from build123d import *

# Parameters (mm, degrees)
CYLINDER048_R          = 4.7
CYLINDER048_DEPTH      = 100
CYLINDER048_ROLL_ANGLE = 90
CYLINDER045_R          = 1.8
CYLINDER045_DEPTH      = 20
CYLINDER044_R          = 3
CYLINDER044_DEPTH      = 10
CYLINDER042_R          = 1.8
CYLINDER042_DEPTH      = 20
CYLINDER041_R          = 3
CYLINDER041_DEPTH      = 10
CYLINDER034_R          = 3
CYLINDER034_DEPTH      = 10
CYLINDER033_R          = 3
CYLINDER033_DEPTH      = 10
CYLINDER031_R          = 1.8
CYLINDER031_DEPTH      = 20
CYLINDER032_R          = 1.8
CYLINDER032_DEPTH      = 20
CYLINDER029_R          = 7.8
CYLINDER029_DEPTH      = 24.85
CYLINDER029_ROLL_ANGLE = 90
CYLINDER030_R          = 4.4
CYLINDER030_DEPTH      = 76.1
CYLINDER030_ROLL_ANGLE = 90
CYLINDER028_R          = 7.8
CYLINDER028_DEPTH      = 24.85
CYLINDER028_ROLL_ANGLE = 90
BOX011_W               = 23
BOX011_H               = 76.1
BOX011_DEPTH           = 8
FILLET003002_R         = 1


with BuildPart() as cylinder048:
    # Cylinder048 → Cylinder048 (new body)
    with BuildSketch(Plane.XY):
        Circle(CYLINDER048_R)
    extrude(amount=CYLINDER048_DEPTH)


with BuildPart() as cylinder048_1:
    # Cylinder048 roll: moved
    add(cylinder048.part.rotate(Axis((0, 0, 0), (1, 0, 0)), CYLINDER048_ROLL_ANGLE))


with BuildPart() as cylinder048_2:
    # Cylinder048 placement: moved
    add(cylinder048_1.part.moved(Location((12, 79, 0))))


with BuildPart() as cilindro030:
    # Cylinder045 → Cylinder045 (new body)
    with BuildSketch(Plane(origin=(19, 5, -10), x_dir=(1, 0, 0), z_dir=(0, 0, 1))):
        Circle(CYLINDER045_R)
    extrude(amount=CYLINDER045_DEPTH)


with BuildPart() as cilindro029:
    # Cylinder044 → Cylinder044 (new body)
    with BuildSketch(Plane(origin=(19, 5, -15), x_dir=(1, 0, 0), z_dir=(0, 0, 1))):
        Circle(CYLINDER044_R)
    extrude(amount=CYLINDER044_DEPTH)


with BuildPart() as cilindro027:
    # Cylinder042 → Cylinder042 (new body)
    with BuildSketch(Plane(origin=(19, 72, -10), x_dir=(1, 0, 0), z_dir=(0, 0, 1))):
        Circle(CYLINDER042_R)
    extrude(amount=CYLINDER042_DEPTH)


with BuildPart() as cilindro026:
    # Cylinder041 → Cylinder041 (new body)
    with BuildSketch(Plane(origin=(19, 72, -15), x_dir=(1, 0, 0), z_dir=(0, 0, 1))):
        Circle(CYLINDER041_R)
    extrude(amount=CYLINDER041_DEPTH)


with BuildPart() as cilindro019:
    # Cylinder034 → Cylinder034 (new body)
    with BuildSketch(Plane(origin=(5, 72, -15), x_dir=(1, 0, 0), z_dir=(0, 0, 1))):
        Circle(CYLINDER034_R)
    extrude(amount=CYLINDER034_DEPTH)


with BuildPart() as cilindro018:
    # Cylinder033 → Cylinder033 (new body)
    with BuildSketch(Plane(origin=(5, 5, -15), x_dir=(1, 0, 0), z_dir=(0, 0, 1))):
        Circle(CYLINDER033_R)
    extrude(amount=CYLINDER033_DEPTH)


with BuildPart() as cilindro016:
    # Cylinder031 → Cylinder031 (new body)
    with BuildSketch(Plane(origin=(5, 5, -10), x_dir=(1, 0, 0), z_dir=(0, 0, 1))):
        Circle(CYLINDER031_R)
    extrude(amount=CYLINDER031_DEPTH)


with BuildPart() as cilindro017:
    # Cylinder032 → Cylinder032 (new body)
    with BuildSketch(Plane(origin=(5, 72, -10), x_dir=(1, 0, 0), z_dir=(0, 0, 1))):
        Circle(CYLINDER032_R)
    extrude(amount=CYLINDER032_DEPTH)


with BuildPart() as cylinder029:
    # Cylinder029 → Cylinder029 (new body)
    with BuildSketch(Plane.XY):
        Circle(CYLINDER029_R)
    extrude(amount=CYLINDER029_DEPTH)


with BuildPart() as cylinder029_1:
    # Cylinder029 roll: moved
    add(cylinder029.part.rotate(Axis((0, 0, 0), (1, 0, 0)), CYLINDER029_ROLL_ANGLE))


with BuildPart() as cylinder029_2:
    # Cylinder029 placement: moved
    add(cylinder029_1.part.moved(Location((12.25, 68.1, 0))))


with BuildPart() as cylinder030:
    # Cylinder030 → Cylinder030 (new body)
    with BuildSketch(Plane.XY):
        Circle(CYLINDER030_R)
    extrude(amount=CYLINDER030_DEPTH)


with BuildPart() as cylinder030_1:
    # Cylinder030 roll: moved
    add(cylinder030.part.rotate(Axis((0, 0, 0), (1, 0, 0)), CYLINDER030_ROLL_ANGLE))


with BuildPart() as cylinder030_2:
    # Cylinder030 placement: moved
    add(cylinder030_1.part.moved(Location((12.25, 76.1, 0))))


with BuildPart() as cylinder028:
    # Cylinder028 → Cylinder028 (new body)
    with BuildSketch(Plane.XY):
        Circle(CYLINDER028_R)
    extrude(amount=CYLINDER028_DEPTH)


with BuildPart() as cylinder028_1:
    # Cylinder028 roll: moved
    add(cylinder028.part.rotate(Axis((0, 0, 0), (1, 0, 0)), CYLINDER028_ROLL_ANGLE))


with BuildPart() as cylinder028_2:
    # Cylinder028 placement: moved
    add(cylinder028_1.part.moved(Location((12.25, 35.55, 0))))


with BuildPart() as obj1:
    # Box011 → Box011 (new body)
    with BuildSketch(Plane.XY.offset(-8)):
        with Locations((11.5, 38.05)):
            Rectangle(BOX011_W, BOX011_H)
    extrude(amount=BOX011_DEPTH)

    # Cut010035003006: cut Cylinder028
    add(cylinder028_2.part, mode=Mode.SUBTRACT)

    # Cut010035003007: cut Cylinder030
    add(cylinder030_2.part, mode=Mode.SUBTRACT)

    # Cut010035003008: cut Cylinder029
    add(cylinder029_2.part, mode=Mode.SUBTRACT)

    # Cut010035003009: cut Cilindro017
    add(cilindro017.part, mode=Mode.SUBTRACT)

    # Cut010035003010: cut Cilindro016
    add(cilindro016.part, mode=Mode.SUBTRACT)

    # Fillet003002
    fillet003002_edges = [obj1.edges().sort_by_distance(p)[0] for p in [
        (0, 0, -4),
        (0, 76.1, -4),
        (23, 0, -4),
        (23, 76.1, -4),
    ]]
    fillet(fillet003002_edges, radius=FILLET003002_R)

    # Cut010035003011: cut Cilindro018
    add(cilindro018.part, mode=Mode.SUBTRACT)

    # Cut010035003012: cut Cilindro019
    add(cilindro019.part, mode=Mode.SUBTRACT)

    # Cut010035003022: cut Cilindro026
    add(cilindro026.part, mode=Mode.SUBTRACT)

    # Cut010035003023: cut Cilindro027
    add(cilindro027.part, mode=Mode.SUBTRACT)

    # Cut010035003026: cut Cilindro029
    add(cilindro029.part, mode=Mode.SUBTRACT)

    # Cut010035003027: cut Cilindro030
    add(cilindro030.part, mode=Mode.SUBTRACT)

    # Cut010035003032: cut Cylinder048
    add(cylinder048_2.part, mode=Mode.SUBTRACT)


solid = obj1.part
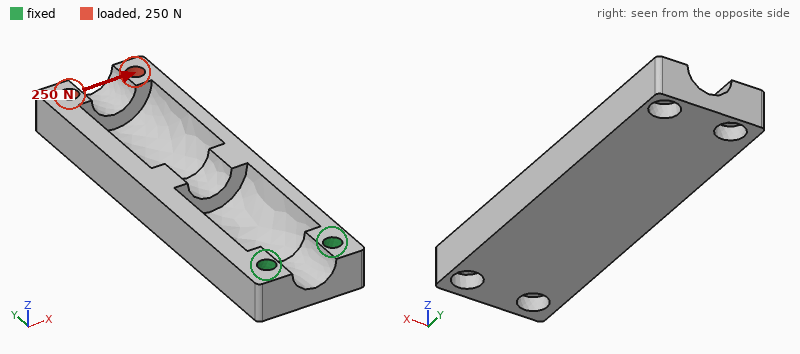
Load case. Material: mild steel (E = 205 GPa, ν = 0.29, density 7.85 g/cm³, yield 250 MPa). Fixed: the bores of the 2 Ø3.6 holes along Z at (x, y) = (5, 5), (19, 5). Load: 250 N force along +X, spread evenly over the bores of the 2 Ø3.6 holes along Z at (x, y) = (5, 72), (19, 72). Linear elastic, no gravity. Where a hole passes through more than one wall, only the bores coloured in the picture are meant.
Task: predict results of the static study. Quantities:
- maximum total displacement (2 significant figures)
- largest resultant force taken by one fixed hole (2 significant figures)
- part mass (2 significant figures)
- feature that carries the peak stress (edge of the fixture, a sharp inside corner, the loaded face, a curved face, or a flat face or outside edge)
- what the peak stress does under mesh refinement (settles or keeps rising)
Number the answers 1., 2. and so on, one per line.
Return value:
1. 60 µm
2. 900 N
3. 61 g
4. edge of the fixture
5. keeps rising
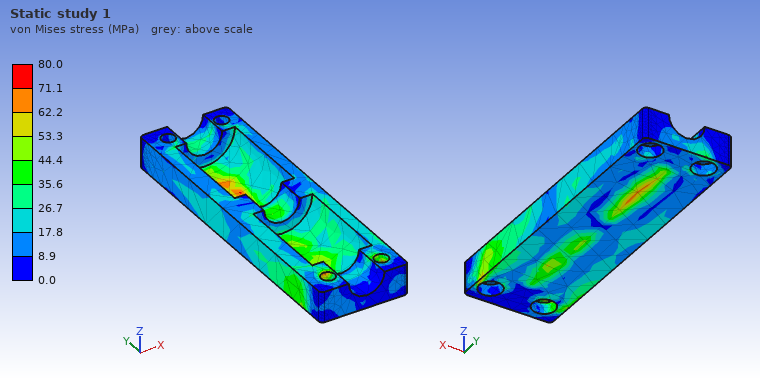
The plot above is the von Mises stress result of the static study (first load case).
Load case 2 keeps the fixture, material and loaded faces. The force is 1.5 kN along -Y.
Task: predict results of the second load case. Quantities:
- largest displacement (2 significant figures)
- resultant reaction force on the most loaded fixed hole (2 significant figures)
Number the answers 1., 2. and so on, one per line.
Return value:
1. 84 µm
2. 750 N
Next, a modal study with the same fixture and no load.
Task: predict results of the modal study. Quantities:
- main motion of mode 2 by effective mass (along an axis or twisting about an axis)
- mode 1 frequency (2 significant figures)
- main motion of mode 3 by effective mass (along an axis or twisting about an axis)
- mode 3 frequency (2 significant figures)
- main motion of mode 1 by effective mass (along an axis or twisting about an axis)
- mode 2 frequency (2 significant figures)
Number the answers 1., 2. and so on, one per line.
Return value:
1. along X
2. 1200 Hz
3. along X
4. 4500 Hz
5. along Z
6. 2600 Hz
